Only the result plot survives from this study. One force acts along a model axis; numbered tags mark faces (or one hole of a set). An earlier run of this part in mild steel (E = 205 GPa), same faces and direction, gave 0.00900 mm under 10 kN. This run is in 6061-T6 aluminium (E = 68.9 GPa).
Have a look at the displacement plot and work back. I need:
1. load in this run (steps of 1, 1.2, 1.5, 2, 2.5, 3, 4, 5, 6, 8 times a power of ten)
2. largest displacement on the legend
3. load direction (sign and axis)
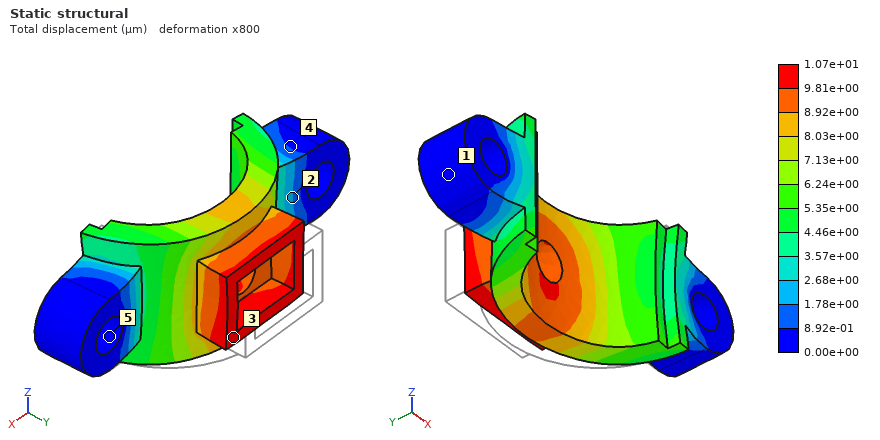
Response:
4 kN
1.07e+01 µm
-Y
